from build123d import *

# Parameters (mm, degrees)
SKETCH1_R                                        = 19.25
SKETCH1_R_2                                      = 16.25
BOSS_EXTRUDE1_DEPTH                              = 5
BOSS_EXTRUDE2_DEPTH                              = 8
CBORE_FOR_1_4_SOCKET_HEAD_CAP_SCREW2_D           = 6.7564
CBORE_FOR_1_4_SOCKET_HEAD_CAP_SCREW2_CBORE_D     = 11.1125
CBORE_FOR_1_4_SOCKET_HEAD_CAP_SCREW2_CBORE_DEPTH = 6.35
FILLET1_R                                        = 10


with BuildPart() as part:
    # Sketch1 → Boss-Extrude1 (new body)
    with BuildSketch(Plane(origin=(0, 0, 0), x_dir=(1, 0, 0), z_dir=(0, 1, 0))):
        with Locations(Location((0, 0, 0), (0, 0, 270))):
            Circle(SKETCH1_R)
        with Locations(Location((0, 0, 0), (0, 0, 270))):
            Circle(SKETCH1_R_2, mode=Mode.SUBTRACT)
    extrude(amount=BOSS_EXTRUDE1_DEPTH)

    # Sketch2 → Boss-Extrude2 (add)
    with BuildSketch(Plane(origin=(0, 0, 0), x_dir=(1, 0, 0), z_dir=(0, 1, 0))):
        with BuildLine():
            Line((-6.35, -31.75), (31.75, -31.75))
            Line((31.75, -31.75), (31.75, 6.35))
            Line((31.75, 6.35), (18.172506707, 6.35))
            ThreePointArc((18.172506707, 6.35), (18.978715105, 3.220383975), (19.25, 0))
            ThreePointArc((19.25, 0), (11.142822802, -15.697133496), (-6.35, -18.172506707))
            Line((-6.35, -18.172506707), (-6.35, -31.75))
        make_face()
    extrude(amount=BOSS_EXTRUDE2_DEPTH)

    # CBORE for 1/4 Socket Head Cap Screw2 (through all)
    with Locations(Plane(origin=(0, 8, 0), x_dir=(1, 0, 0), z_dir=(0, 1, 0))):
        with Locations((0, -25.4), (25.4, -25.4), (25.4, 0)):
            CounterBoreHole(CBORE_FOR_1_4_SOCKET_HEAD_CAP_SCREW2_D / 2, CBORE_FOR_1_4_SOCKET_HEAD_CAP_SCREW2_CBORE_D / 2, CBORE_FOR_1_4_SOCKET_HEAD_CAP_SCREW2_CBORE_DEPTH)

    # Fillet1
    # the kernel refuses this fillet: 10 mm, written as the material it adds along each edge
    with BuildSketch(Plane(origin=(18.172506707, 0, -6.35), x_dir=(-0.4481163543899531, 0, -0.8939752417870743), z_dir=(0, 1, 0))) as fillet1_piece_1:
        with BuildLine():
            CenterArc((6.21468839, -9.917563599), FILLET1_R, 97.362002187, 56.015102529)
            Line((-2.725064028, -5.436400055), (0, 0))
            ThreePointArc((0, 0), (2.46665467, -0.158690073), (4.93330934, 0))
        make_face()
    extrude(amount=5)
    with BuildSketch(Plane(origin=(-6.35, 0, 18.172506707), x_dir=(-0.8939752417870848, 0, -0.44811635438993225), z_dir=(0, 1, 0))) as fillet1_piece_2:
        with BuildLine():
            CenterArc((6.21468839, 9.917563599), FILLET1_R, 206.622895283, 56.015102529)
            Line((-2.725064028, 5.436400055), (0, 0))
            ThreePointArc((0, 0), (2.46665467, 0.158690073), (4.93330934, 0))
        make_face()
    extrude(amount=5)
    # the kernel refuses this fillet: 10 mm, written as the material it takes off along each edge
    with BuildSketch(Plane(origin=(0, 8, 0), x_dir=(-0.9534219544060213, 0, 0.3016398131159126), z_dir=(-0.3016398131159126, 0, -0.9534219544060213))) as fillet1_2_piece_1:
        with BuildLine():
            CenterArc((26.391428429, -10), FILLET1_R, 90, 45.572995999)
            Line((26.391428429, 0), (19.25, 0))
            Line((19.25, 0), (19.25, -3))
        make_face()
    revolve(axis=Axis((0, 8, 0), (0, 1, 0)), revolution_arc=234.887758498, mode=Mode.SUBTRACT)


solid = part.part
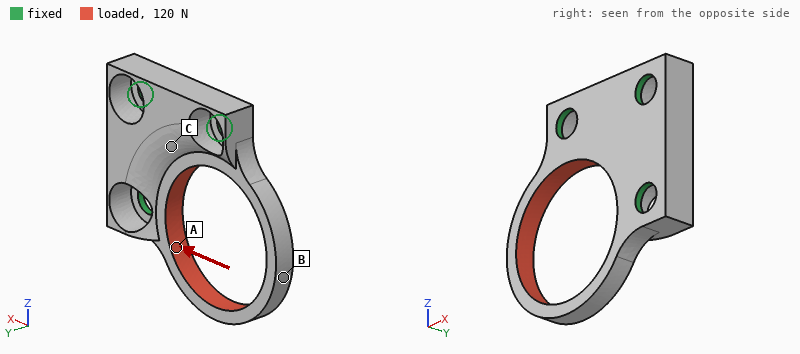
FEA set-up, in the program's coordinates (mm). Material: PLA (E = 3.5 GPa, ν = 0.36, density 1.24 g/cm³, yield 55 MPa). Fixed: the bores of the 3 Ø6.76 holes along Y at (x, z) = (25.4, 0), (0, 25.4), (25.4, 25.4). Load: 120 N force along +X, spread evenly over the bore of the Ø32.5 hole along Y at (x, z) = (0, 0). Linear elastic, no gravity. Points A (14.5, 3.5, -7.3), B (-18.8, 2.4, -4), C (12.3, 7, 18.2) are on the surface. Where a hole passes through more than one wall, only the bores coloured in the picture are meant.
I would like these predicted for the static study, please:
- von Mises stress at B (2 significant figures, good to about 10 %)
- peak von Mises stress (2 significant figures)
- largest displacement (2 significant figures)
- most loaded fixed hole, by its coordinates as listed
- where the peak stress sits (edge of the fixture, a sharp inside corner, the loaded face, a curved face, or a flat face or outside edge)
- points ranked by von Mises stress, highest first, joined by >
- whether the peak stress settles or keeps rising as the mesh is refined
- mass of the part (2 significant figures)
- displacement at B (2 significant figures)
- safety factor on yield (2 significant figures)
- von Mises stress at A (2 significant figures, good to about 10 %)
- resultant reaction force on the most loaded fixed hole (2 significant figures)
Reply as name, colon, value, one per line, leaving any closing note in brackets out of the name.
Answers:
von Mises stress at B: 12 MPa
peak von Mises stress: 26 MPa
largest displacement: 0.51 mm
most loaded fixed hole, by its coordinates as listed: (25.4, 0)
where the peak stress sits: a curved face
points ranked by von Mises stress, highest first, joined by >: A > B > C
whether the peak stress settles or keeps rising as the mesh is refined: settles
mass of the part: 8.1 g
displacement at B: 0.49 mm
safety factor on yield: 2.1
von Mises stress at A: 20 MPa
resultant reaction force on the most loaded fixed hole: 82 N
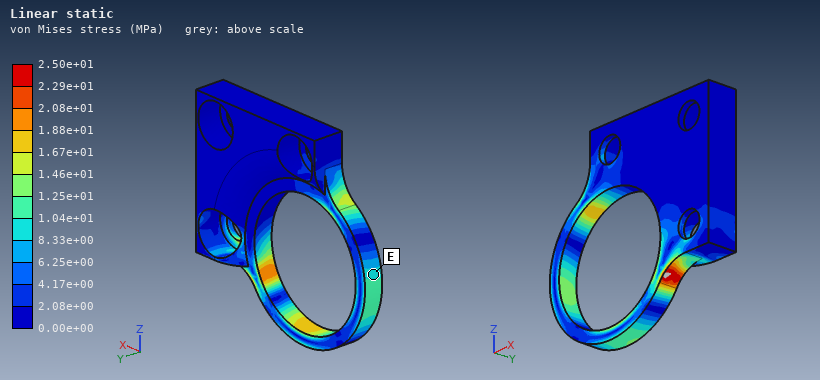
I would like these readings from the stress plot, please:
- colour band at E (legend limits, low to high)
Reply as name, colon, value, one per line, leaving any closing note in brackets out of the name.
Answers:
colour band at E: 8.33e+00 to 1.04e+01 MPa
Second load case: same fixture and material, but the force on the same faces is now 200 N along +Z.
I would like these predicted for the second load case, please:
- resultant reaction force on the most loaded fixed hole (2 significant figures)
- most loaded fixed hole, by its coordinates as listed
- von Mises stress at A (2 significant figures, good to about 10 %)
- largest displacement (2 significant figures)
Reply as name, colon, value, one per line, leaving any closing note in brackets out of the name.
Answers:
resultant reaction force on the most loaded fixed hole: 140 N
most loaded fixed hole, by its coordinates as listed: (0, 25.4)
von Mises stress at A: 29 MPa
largest displacement: 0.85 mm
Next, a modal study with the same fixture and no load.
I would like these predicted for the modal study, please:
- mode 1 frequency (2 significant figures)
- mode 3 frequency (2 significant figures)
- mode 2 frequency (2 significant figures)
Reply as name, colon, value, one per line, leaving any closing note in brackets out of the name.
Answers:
mode 1 frequency: 880 Hz
mode 3 frequency: 2200 Hz
mode 2 frequency: 1600 Hz
